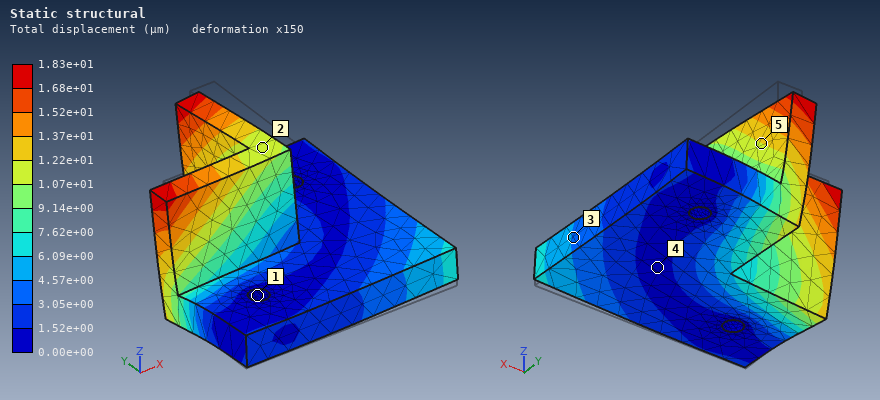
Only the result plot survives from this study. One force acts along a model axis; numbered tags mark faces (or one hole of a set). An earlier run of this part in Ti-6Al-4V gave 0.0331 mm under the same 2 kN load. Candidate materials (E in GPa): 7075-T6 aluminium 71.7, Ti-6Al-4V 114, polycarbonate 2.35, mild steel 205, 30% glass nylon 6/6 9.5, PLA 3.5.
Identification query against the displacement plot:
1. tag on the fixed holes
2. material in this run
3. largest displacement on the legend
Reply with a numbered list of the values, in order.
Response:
1. 1
2. mild steel
3. 1.83e+01 µm
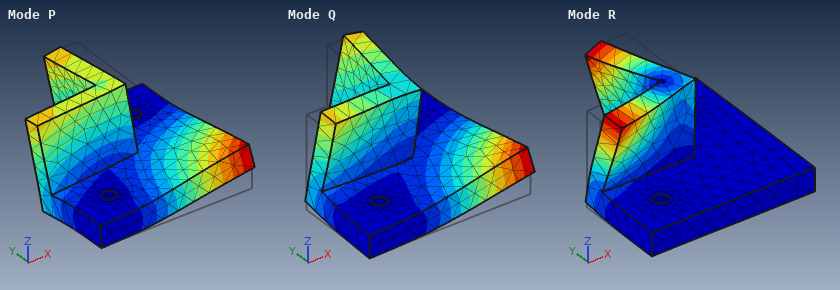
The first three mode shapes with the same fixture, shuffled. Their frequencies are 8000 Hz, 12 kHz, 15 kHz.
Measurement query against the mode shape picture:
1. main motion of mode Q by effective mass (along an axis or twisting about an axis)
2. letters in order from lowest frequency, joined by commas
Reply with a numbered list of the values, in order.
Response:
1. along Z
2. P, Q, R
